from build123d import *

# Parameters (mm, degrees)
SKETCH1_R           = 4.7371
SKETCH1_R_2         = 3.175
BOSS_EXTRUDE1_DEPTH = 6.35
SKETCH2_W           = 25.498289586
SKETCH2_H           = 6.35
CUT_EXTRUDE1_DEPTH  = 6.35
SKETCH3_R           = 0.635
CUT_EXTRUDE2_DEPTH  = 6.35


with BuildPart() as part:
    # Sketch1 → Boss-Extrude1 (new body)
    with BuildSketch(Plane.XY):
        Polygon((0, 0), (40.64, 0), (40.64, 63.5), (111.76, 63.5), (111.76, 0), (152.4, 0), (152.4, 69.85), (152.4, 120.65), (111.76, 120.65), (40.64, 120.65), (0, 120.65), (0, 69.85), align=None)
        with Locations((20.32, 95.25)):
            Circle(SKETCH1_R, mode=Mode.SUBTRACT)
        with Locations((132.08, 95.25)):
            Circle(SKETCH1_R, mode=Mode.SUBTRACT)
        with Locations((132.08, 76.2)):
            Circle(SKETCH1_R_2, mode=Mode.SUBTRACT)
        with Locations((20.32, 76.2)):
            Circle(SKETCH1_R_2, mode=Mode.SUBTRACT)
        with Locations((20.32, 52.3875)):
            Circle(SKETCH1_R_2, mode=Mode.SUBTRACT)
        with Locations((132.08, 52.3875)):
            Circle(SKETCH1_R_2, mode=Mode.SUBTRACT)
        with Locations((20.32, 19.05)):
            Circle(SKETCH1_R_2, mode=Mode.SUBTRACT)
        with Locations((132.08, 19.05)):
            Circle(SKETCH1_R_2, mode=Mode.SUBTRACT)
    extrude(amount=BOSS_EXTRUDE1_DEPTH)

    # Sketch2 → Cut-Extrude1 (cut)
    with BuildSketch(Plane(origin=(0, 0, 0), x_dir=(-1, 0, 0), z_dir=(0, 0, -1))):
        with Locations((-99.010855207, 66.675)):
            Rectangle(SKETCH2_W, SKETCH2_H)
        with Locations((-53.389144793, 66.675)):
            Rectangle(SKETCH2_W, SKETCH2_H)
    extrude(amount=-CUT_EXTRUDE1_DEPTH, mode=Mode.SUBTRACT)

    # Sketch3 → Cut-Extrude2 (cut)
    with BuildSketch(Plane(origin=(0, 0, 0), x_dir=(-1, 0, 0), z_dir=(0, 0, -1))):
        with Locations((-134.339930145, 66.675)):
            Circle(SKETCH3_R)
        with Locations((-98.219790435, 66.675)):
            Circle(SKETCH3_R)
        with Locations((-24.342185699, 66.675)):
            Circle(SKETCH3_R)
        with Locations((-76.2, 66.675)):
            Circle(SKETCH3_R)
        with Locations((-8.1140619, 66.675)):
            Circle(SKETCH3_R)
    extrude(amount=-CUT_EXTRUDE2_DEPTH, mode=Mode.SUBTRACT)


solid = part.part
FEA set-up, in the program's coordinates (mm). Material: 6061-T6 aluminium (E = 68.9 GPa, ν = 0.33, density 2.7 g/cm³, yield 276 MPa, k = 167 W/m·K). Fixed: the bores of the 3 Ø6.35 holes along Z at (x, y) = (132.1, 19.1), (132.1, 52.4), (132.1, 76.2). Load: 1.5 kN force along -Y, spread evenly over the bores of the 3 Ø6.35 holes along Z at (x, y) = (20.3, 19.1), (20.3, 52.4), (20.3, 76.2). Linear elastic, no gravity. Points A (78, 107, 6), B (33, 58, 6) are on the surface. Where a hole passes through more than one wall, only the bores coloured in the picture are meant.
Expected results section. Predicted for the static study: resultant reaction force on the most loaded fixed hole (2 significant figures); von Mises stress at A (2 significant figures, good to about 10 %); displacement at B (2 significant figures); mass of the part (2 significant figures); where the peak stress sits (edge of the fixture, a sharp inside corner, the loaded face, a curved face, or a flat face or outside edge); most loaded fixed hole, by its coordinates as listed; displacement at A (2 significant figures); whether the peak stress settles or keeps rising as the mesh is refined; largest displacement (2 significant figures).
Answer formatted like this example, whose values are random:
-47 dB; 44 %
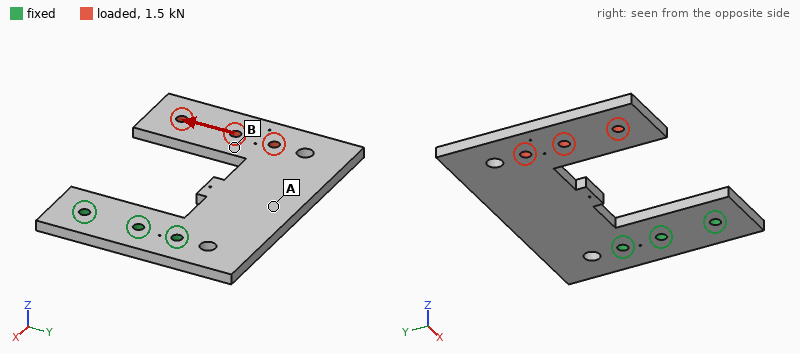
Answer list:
4.4 kN; 17 MPa; 0.32 mm; 230 g; edge of the fixture; (132.1, 76.2); 0.16 mm; keeps rising; 0.54 mm
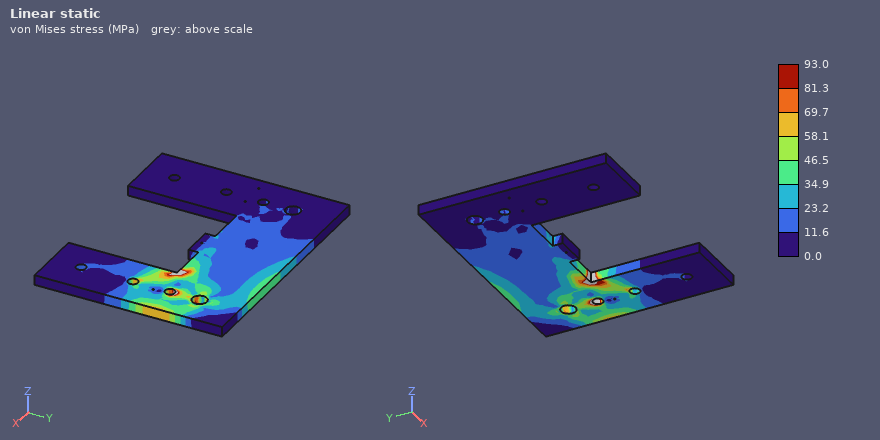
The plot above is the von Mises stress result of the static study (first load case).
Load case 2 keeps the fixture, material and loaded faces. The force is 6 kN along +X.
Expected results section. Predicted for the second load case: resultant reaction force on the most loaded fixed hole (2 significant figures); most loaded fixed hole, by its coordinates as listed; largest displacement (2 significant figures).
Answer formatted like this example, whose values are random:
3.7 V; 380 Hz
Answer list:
4.1 kN; (132.1, 52.4); 1.1 mm
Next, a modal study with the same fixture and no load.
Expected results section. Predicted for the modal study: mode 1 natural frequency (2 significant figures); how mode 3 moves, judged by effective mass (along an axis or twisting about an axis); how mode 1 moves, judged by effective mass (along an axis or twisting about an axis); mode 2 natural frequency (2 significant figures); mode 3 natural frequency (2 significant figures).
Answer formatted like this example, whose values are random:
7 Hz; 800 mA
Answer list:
190 Hz; along Y; along Z; 420 Hz; 960 Hz
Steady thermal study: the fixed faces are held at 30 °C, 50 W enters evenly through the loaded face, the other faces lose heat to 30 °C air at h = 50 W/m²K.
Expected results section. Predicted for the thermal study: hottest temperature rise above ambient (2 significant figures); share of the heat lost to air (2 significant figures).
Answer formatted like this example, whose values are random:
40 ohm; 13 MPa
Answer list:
61 K; 73 %
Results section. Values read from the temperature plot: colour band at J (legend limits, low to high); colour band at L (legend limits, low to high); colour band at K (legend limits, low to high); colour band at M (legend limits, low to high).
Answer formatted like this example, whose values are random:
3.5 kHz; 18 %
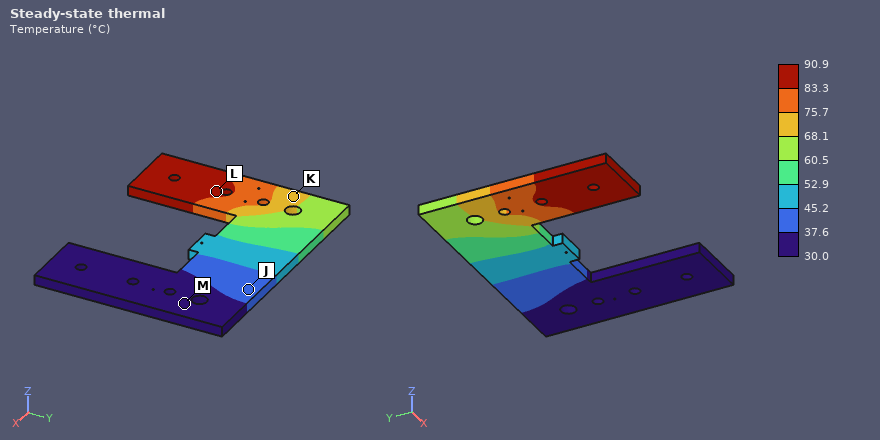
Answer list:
37.6 to 45.2 °C; 83.3 to 90.9 °C; 68.1 to 75.7 °C; 30.0 to 37.6 °C
